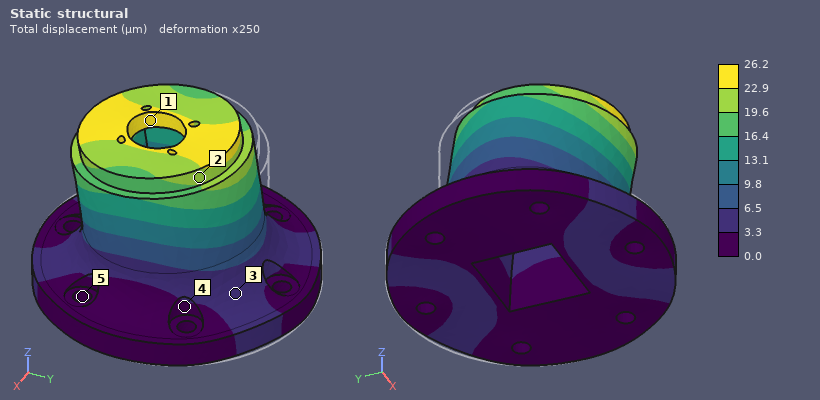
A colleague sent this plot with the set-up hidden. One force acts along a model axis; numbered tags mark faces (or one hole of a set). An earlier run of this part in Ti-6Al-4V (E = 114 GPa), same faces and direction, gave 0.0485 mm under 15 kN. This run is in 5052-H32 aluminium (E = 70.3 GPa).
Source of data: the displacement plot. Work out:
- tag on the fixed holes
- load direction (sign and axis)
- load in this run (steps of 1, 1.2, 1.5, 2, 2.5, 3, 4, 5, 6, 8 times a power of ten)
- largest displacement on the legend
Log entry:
5
-Y
5 kN
26.2 µm
